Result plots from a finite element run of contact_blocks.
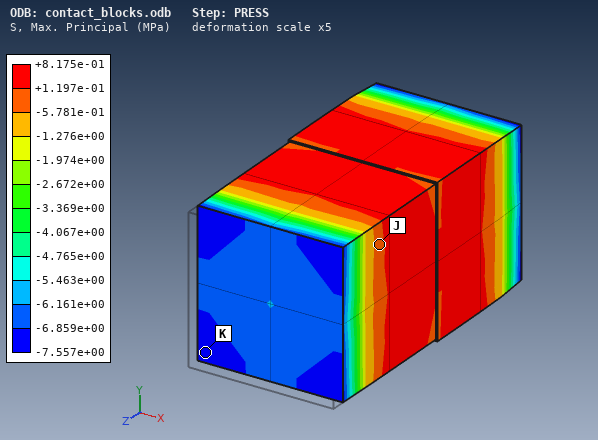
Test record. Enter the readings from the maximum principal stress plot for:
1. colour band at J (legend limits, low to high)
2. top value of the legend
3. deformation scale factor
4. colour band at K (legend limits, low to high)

-5.781e-01 to +1.197e-01 MPa
+8.175e-01 MPa
5
-7.557e+00 to -6.859e+00 MPa
